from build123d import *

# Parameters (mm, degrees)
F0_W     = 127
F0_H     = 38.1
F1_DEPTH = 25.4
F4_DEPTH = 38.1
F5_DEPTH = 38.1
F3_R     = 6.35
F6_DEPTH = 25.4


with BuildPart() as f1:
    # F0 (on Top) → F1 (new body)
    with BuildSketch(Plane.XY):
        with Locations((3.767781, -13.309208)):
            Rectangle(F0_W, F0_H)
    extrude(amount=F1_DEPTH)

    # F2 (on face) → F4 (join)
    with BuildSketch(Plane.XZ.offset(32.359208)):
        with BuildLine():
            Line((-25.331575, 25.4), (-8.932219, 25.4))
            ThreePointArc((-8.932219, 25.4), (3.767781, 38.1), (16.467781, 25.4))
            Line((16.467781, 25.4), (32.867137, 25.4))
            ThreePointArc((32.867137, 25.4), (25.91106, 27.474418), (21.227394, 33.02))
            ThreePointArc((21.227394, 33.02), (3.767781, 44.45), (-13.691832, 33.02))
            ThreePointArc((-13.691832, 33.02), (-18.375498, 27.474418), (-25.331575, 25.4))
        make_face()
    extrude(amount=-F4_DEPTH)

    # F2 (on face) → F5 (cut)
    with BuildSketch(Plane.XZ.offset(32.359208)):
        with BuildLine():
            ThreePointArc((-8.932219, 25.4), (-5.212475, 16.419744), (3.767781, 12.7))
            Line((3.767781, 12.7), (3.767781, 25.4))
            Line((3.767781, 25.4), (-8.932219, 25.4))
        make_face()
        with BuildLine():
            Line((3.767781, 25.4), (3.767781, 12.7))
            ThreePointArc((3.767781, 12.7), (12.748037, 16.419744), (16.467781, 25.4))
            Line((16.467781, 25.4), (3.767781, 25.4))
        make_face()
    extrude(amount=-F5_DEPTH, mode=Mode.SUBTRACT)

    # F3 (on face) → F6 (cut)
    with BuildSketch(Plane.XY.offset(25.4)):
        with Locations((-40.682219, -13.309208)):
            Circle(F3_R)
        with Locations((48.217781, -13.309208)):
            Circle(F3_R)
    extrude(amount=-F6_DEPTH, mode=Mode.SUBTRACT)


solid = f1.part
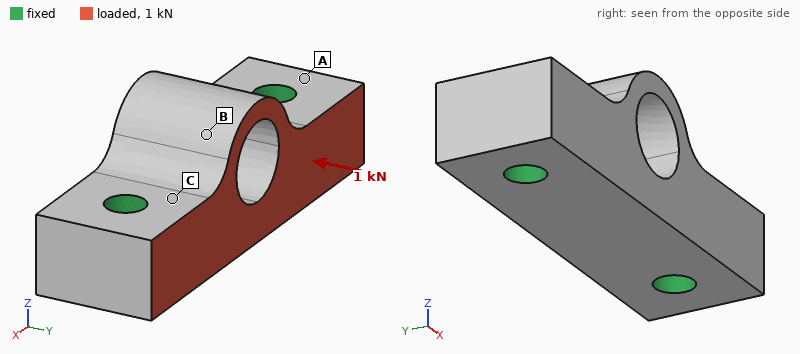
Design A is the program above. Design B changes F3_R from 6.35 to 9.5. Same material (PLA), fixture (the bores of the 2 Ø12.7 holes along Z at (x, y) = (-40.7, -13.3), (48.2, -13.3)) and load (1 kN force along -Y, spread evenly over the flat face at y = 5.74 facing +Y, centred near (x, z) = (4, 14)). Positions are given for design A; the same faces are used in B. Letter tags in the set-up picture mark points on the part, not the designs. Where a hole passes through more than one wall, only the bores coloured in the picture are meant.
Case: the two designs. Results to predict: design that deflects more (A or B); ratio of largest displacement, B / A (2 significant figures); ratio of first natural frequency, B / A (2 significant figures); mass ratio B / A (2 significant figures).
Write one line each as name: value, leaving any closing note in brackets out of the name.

design that deflects more: A
ratio of largest displacement, B / A: 0.78
ratio of first natural frequency, B / A: 1.2
mass ratio B / A: 0.93
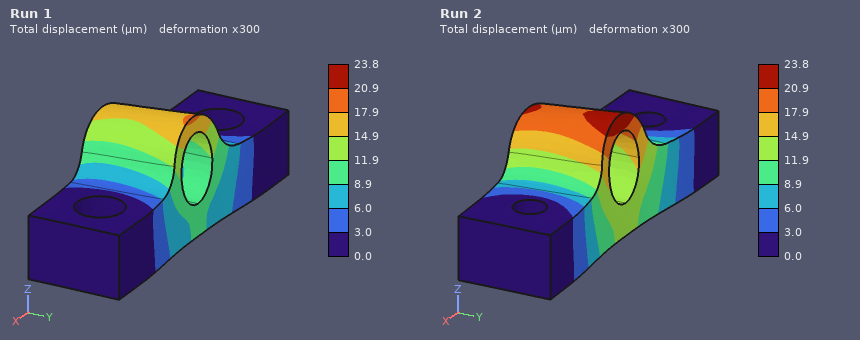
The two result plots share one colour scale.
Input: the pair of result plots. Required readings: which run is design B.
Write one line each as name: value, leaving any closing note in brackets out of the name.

which run is design B: Run 1
